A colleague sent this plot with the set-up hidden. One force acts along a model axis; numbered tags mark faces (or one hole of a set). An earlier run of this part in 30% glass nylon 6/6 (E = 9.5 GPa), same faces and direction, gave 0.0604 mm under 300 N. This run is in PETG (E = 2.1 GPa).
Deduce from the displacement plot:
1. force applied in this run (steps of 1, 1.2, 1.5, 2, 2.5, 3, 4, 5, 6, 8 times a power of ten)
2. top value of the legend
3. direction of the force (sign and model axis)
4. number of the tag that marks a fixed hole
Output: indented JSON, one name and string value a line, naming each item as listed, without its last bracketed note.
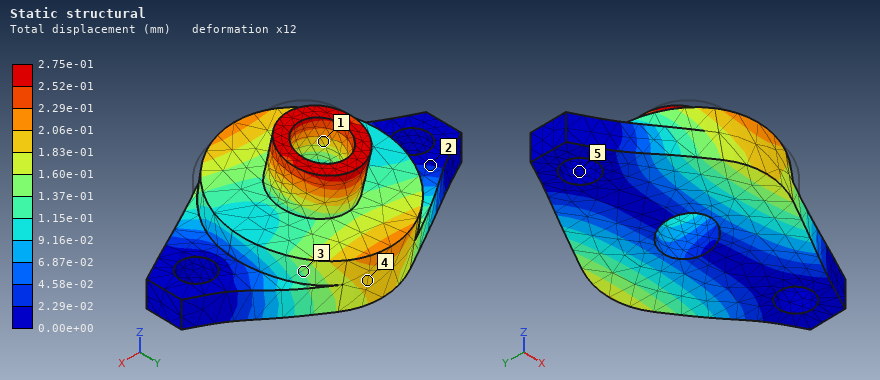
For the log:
{
  "force applied in this run": "300 N",
  "top value of the legend": "2.75e-01 mm",
  "direction of the force": "+Y",
  "number of the tag that marks a fixed hole": "5"
}
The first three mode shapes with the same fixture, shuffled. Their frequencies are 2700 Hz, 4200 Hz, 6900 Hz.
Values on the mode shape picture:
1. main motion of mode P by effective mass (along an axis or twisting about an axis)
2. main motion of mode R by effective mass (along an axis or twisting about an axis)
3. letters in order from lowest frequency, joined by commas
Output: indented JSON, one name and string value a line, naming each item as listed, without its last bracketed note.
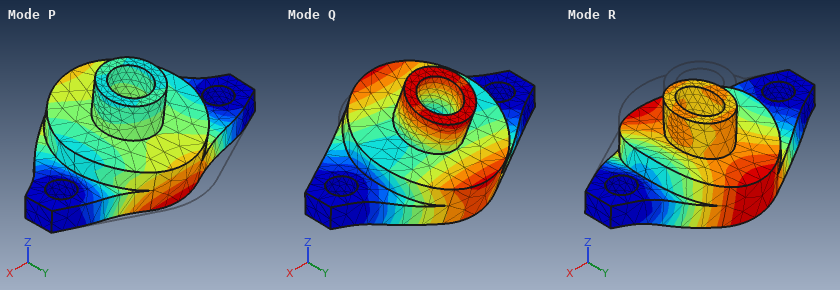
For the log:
{
  "main motion of mode P by effective mass": "along Y",
  "main motion of mode R by effective mass": "along Z",
  "letters in order from lowest frequency, joined by commas": "Q, R, P"
}
